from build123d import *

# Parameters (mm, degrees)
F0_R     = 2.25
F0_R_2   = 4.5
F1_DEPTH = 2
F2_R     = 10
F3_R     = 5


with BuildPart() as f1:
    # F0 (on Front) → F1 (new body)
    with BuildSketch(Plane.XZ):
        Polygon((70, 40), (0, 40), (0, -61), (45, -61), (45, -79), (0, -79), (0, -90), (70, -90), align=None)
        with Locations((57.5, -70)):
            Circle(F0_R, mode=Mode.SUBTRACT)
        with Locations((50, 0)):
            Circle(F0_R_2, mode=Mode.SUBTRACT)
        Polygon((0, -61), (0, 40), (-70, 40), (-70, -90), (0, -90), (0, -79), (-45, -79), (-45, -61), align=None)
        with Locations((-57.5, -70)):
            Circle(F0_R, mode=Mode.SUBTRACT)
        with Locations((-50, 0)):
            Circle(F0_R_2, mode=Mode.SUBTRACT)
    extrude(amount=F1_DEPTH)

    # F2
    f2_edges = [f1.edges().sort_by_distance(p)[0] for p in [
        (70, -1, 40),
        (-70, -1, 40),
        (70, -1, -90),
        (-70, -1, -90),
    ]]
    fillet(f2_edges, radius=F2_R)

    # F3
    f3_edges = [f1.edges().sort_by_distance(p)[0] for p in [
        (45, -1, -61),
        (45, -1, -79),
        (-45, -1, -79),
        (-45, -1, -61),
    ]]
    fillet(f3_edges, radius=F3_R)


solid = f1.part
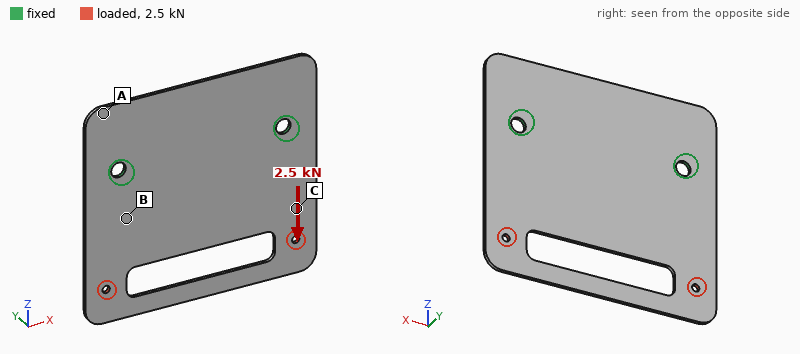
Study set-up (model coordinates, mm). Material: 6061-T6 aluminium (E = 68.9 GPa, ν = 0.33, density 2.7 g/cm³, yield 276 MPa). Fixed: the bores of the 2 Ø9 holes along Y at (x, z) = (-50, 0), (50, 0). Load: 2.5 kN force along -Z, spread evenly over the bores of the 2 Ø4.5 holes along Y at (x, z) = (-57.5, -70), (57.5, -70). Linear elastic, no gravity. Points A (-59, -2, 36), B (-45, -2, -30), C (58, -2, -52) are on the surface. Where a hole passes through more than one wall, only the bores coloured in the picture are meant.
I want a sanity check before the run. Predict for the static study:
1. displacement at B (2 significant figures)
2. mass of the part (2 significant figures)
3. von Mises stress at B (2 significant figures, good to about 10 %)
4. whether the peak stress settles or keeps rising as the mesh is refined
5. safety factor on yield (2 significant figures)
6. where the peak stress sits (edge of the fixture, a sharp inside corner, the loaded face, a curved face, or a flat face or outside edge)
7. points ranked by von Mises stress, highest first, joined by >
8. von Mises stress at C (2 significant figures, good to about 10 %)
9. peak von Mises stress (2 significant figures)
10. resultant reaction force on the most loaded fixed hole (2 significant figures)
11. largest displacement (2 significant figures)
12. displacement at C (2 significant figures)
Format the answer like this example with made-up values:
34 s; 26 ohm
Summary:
7.2 µm; 88 g; 15 MPa; settles; 3.3; the loaded face; C > B > A; 23 MPa; 84 MPa; 1.3 kN; 25 µm; 15 µm
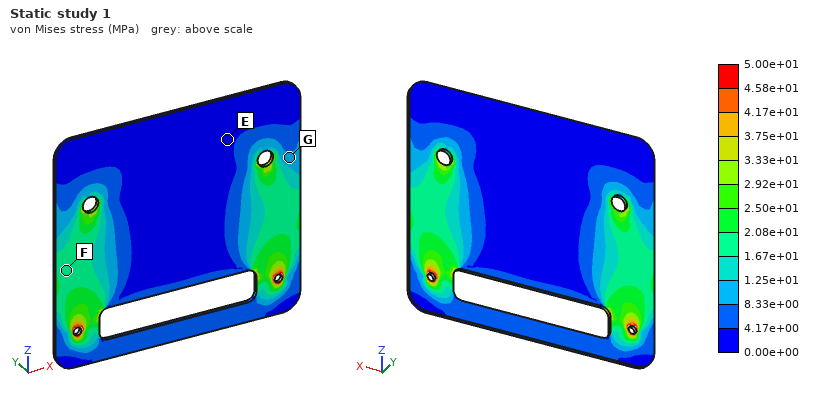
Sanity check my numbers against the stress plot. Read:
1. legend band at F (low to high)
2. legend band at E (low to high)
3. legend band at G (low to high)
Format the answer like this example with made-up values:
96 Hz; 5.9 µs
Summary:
1.67e+01 to 2.08e+01 MPa; 0.00e+00 to 4.17e+00 MPa; 8.33e+00 to 1.25e+01 MPa
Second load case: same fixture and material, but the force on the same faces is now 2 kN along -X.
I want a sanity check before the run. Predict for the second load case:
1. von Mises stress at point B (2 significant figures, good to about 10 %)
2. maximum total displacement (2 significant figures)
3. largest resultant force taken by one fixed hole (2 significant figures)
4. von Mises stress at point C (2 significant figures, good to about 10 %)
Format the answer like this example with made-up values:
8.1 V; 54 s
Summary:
7.9 MPa; 96 µm; 1.7 kN; 16 MPa
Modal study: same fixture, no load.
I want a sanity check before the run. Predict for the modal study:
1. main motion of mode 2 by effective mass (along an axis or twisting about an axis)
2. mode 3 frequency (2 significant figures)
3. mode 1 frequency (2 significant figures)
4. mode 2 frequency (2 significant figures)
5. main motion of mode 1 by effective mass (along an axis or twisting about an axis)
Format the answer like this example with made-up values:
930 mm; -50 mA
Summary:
twisting about Z; 730 Hz; 220 Hz; 370 Hz; along Y
